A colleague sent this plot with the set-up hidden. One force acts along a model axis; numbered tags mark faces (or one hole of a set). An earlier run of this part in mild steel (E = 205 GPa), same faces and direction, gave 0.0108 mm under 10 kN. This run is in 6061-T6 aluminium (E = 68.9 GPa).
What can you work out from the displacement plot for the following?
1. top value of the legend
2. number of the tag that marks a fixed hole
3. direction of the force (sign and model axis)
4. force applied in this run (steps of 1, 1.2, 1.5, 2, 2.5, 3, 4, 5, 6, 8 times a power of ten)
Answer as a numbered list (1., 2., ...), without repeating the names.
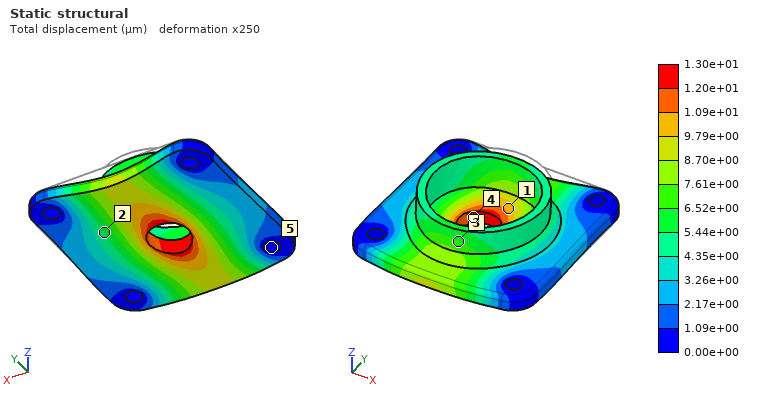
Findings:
1. 1.30e+01 µm
2. 5
3. -Y
4. 4 kN
